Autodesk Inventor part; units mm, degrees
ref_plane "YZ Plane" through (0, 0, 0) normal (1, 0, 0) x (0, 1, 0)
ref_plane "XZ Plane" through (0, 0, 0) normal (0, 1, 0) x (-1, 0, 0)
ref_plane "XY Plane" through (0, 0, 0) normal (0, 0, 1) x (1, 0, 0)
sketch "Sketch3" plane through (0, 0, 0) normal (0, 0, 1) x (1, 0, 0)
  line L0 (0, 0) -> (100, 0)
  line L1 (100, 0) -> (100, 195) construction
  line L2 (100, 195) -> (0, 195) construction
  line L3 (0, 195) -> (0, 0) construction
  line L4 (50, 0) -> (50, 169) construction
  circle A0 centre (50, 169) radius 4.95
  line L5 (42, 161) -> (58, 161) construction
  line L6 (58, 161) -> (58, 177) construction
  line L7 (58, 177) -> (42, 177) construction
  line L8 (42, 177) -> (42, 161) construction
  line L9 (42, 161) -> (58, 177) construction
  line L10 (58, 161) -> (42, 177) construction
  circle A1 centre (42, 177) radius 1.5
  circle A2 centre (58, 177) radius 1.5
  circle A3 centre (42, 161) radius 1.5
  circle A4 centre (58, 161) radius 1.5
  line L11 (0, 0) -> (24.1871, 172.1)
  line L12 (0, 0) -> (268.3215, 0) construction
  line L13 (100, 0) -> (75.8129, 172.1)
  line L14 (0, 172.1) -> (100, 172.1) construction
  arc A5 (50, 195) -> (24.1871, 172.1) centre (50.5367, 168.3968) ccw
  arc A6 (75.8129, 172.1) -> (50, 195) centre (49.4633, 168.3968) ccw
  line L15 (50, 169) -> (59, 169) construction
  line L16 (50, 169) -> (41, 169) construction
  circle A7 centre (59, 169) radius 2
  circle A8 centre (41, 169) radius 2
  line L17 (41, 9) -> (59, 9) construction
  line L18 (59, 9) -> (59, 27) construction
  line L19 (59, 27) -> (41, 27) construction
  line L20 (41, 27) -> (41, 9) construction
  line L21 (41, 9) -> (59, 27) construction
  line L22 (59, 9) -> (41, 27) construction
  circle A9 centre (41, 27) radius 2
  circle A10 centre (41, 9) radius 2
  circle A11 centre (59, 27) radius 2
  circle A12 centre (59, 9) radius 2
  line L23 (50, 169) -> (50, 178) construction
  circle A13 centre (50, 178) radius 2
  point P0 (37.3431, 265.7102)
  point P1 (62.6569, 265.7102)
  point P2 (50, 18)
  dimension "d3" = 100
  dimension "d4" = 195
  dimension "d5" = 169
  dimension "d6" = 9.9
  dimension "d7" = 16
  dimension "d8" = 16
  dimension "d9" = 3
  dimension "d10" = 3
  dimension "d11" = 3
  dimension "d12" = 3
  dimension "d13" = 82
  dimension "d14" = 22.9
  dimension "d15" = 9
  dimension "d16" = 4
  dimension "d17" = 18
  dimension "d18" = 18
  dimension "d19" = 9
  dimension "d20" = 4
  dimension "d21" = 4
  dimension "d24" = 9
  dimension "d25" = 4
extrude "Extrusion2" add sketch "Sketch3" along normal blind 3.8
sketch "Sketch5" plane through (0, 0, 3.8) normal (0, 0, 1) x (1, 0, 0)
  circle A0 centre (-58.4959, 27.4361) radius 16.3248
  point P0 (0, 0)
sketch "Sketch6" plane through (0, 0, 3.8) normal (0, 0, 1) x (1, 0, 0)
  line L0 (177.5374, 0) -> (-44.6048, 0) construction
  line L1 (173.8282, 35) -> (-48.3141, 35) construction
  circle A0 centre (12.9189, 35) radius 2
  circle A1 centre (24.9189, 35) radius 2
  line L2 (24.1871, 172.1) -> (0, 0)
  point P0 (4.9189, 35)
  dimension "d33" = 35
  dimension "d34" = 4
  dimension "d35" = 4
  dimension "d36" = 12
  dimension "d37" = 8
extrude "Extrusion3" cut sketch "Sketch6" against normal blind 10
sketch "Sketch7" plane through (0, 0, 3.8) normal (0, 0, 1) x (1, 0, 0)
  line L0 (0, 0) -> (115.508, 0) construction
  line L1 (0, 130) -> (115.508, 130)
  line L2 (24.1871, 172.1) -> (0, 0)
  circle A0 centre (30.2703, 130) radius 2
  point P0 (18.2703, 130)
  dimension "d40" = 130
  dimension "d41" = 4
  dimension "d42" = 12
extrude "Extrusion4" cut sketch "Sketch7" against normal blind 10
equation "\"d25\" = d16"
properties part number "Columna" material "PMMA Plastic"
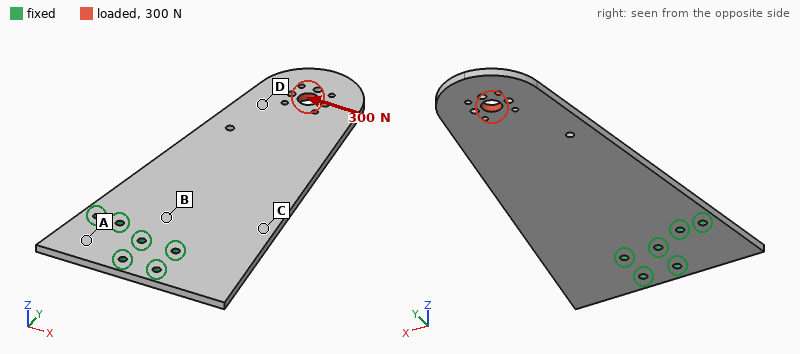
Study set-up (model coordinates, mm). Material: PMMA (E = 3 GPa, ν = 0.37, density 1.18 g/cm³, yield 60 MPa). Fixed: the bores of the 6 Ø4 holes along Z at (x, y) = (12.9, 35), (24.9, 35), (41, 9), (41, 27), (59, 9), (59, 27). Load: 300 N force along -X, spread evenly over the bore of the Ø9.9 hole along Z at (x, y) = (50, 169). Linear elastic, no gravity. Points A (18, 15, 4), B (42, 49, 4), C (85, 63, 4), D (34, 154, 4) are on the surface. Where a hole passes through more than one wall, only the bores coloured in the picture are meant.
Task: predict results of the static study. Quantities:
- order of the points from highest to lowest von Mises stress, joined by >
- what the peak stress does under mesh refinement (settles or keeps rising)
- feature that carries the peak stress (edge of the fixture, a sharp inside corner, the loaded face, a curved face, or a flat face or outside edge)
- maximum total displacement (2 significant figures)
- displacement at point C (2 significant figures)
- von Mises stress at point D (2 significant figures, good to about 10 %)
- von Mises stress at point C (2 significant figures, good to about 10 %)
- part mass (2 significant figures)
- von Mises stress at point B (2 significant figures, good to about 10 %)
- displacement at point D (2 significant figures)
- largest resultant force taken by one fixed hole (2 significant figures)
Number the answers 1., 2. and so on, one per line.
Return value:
1. C > B > D > A
2. keeps rising
3. edge of the fixture
4. 1.1 mm
5. 0.21 mm
6. 2.5 MPa
7. 5.5 MPa
8. 61 g
9. 3.5 MPa
10. 0.76 mm
11. 570 N
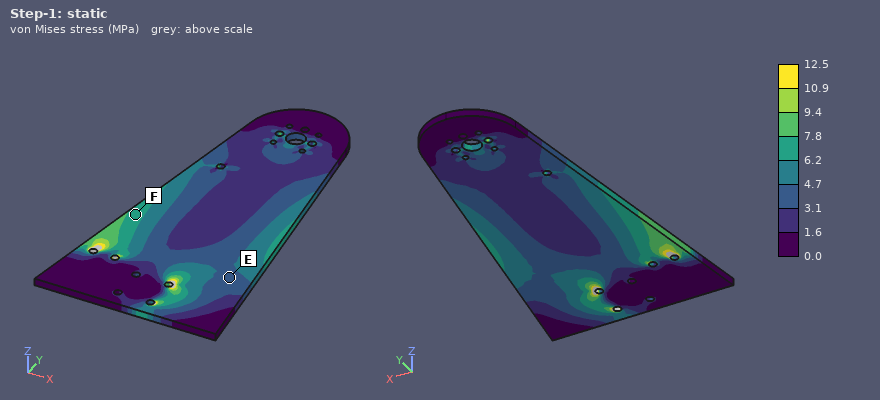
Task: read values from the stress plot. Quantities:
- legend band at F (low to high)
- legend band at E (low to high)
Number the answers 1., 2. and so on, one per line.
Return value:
1. 6.2 to 7.8 MPa
2. 3.1 to 4.7 MPa
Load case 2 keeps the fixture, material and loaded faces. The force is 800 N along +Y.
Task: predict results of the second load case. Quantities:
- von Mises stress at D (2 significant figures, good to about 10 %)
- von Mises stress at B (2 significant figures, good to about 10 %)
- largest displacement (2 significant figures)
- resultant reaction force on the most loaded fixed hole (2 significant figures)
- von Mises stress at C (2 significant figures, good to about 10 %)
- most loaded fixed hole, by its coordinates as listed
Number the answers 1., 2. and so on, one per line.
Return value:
1. 3.7 MPa
2. 3.1 MPa
3. 0.24 mm
4. 350 N
5. 2.1 MPa
6. (59, 27)
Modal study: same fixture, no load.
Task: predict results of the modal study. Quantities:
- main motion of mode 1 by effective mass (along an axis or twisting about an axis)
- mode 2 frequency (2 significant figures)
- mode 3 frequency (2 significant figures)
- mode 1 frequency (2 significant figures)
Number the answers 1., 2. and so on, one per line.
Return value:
1. along Z
2. 230 Hz
3. 270 Hz
4. 48 Hz
